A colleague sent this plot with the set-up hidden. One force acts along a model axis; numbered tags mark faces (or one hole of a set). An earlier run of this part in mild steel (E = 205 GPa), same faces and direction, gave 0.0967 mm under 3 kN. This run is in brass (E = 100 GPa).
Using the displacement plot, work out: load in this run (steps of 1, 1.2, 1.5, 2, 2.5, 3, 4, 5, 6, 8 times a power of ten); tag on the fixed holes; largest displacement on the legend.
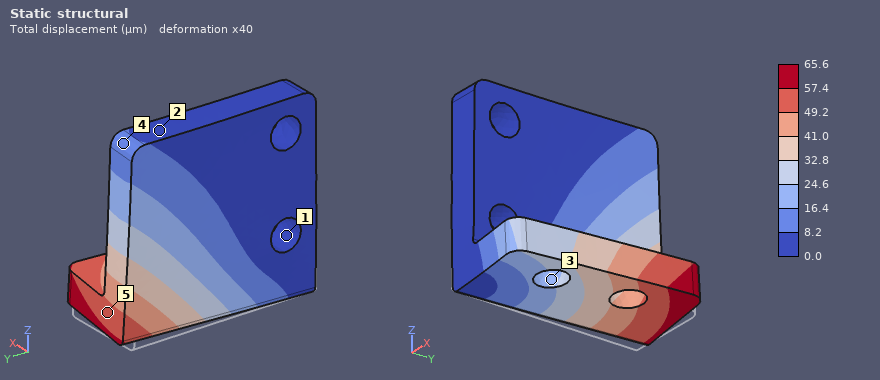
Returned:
1 kN
1
65.6 µm
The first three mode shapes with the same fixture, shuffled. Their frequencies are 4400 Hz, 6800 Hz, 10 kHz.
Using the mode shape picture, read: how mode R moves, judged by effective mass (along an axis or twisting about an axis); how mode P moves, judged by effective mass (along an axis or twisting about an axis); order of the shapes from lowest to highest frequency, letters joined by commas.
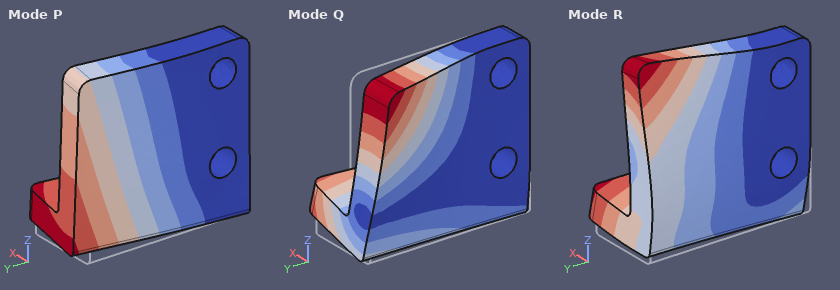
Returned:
along Z
along X
P, Q, R
